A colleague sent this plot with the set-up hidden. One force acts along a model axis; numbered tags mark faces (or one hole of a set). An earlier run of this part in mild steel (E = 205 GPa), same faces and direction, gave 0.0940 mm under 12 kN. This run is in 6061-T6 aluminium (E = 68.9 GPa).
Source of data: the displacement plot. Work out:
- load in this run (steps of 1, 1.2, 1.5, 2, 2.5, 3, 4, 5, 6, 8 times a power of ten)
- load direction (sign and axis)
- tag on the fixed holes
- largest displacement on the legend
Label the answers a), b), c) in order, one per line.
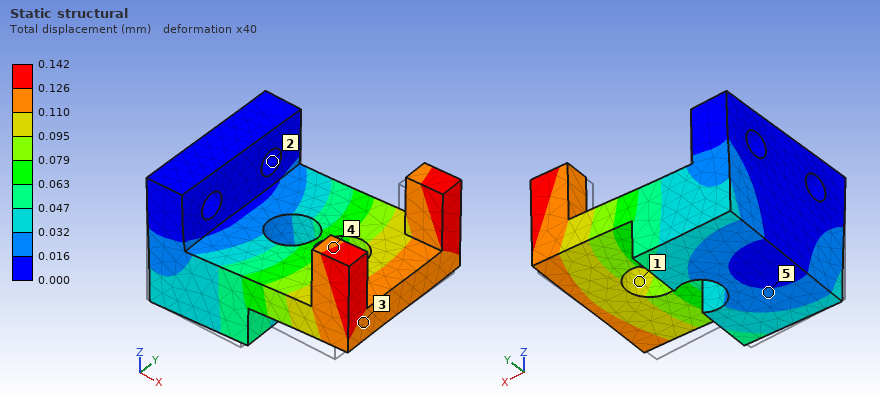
a) 6 kN
b) +Y
c) 2
d) 0.142 mm
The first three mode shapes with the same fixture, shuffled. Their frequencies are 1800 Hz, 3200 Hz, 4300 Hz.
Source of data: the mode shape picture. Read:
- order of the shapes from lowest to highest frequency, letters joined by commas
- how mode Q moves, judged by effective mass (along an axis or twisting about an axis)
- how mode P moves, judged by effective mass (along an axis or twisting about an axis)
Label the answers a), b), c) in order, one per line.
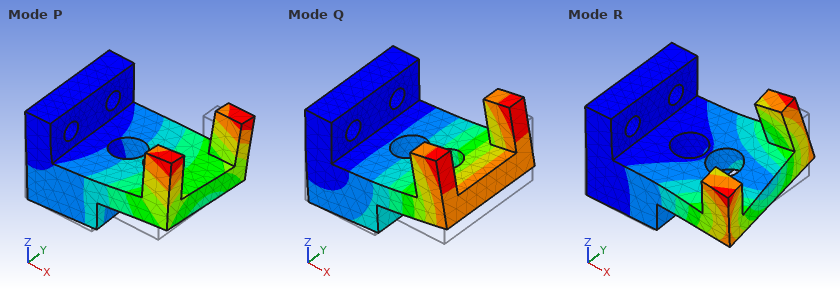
a) Q, P, R
b) along Z
c) along Y
